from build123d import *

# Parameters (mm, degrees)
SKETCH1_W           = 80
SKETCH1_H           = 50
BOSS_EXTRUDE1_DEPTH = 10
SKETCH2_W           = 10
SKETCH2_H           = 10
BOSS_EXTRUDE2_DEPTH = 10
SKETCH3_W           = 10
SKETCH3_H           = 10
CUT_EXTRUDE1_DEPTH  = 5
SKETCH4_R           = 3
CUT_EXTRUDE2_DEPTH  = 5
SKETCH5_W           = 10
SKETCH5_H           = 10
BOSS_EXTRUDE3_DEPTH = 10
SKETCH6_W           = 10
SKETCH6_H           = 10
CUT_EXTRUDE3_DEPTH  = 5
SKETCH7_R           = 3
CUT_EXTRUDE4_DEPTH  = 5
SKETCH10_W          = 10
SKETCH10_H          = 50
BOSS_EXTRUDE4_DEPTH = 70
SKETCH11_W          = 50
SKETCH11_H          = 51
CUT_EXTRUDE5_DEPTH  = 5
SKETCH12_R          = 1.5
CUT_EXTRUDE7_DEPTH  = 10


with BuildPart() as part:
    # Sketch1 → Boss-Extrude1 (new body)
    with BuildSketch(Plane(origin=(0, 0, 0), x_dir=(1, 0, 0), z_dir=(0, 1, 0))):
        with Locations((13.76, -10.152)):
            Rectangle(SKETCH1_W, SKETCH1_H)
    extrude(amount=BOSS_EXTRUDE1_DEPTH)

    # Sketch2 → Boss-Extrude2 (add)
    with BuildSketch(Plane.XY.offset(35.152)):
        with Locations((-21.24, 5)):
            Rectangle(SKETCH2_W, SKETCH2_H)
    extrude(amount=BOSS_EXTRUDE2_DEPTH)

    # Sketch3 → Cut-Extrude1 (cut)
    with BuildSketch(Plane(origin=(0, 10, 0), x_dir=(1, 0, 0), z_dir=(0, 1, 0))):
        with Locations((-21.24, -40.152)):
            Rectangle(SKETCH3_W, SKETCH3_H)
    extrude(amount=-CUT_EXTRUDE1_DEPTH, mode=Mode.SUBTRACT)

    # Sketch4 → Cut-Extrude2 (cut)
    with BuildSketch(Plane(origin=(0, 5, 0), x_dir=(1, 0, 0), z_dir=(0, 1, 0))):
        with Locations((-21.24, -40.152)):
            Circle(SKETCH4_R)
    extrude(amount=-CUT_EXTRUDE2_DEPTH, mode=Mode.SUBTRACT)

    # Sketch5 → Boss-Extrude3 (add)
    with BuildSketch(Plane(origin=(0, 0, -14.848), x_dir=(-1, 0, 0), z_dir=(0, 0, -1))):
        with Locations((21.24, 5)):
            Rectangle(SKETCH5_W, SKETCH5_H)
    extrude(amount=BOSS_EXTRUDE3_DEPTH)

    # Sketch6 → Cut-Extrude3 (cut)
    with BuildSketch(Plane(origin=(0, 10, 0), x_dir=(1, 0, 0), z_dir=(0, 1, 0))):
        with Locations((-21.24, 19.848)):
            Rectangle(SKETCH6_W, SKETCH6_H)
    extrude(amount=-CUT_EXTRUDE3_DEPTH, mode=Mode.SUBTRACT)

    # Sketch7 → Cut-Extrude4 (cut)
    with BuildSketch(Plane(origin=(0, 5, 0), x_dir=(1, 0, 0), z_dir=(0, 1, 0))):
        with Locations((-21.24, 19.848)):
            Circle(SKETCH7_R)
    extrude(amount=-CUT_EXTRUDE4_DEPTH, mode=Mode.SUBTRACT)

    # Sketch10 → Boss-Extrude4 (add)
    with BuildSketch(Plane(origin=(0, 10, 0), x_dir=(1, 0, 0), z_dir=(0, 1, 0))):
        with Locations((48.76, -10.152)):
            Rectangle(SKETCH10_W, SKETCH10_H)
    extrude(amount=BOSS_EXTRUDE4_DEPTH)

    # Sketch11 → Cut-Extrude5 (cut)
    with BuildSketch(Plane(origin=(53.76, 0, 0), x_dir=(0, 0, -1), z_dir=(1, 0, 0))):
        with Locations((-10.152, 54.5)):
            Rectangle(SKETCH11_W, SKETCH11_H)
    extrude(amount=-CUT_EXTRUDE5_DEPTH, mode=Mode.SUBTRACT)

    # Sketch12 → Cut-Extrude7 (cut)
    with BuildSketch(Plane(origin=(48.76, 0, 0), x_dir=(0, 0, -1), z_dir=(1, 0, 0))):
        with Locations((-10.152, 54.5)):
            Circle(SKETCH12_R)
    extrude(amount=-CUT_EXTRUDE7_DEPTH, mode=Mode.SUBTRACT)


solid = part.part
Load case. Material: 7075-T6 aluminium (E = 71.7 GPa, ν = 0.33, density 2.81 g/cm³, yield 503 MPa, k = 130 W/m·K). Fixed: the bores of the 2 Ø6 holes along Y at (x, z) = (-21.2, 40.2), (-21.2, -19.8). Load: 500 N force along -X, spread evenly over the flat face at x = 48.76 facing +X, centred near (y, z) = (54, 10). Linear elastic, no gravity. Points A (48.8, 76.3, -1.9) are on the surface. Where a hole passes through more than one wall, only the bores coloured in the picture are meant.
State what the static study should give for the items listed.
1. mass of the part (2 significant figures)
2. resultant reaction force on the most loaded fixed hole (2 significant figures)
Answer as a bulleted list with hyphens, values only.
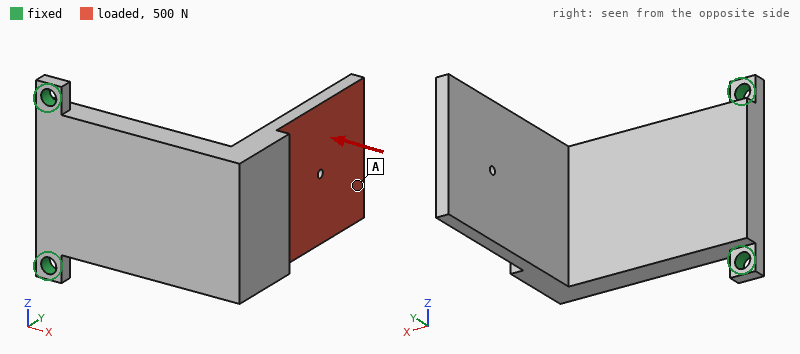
- 180 g
- 250 N
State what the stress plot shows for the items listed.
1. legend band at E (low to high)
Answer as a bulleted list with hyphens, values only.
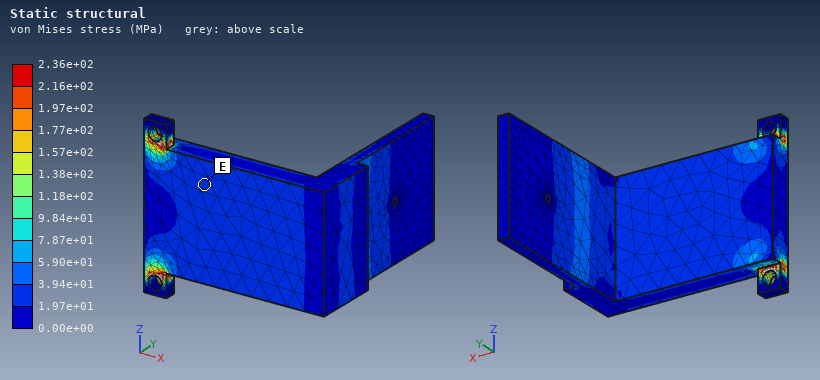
- 1.97e+01 to 3.94e+01 MPa
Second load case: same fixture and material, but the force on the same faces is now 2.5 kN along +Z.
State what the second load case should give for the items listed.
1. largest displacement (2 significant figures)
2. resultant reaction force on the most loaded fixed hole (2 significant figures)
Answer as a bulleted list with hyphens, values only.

- 1.5 mm
- 4.4 kN
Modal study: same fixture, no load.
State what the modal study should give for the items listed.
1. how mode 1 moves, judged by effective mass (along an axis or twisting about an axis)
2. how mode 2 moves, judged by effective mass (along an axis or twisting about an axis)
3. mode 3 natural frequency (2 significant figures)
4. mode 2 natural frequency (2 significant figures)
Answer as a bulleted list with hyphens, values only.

- along Y
- along Z
- 1200 Hz
- 1100 Hz
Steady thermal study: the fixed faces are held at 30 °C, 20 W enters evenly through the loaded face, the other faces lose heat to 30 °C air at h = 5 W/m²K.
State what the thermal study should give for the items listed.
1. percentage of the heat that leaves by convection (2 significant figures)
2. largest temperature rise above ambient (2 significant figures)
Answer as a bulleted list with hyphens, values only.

- 10 %
- 50 K
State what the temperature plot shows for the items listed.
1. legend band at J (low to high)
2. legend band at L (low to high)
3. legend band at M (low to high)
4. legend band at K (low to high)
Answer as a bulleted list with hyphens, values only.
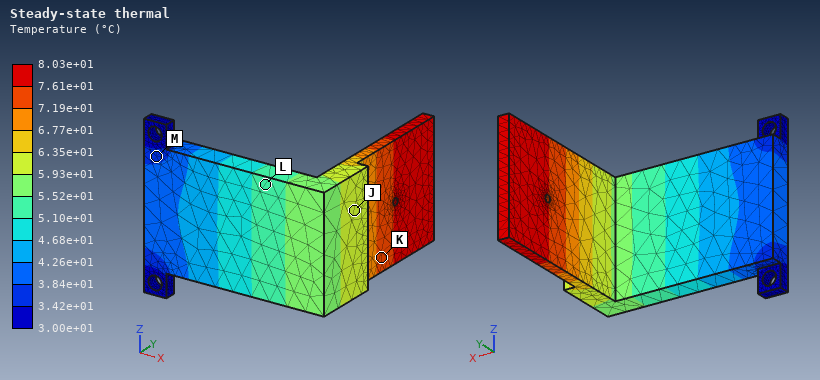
- 5.93e+01 to 6.35e+01 °C
- 5.10e+01 to 5.52e+01 °C
- 3.42e+01 to 3.84e+01 °C
- 7.19e+01 to 7.61e+01 °C
